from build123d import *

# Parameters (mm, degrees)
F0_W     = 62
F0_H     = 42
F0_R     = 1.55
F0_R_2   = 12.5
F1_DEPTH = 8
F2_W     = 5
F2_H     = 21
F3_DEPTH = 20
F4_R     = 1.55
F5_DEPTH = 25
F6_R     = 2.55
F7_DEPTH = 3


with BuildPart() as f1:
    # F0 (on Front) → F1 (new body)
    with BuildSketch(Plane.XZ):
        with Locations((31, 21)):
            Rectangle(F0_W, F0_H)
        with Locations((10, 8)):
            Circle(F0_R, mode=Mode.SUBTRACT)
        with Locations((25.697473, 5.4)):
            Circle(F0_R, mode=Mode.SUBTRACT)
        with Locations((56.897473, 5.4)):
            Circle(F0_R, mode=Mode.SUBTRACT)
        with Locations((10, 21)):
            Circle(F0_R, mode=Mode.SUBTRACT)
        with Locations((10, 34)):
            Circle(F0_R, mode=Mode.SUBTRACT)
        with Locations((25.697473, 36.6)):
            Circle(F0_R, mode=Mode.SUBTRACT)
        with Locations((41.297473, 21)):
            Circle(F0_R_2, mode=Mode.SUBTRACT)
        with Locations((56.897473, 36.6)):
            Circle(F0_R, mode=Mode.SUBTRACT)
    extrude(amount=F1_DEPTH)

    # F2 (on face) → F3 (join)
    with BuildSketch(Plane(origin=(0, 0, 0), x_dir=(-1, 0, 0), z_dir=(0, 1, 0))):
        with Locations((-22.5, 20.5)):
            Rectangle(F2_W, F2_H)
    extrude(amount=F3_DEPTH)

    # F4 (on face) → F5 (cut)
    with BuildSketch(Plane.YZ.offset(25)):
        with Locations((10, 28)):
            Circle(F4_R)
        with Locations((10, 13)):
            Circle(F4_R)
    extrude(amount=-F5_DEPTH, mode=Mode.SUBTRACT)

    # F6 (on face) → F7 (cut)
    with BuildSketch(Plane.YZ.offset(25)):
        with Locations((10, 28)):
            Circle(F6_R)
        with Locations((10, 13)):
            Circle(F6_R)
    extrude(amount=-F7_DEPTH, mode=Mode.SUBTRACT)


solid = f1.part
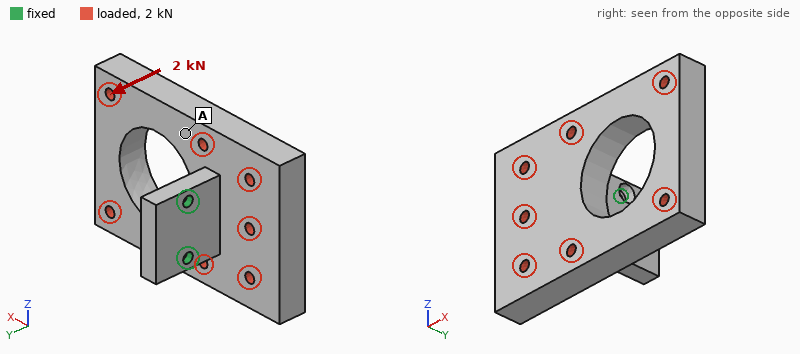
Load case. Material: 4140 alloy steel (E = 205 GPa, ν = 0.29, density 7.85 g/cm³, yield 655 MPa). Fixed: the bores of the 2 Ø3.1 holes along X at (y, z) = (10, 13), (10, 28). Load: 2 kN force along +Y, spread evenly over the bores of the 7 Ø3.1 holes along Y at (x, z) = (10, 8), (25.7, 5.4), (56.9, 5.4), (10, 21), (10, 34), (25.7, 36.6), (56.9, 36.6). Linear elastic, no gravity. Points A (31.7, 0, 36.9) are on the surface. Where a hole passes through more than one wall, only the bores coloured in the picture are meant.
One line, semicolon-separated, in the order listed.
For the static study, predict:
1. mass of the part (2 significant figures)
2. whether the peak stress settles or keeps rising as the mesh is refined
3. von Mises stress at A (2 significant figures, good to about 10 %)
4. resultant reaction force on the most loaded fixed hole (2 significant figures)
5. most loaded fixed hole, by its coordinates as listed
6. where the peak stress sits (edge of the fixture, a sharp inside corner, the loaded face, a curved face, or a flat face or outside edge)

140 g; keeps rising; 54 MPa; 1.1 kN; (10, 28); edge of the fixture
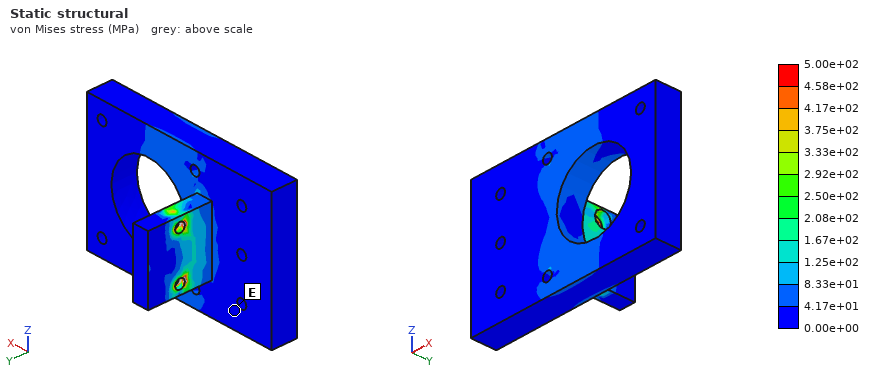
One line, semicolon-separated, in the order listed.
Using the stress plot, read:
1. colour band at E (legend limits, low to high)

0.00e+00 to 4.17e+01 MPa
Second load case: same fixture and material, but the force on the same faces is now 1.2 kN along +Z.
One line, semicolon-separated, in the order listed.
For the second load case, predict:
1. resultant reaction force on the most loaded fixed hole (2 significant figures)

1.3 kN
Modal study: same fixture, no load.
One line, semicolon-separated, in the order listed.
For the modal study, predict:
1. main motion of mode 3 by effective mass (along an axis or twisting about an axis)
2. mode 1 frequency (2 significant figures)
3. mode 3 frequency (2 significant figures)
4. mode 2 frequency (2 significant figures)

along X; 870 Hz; 4400 Hz; 1800 Hz
